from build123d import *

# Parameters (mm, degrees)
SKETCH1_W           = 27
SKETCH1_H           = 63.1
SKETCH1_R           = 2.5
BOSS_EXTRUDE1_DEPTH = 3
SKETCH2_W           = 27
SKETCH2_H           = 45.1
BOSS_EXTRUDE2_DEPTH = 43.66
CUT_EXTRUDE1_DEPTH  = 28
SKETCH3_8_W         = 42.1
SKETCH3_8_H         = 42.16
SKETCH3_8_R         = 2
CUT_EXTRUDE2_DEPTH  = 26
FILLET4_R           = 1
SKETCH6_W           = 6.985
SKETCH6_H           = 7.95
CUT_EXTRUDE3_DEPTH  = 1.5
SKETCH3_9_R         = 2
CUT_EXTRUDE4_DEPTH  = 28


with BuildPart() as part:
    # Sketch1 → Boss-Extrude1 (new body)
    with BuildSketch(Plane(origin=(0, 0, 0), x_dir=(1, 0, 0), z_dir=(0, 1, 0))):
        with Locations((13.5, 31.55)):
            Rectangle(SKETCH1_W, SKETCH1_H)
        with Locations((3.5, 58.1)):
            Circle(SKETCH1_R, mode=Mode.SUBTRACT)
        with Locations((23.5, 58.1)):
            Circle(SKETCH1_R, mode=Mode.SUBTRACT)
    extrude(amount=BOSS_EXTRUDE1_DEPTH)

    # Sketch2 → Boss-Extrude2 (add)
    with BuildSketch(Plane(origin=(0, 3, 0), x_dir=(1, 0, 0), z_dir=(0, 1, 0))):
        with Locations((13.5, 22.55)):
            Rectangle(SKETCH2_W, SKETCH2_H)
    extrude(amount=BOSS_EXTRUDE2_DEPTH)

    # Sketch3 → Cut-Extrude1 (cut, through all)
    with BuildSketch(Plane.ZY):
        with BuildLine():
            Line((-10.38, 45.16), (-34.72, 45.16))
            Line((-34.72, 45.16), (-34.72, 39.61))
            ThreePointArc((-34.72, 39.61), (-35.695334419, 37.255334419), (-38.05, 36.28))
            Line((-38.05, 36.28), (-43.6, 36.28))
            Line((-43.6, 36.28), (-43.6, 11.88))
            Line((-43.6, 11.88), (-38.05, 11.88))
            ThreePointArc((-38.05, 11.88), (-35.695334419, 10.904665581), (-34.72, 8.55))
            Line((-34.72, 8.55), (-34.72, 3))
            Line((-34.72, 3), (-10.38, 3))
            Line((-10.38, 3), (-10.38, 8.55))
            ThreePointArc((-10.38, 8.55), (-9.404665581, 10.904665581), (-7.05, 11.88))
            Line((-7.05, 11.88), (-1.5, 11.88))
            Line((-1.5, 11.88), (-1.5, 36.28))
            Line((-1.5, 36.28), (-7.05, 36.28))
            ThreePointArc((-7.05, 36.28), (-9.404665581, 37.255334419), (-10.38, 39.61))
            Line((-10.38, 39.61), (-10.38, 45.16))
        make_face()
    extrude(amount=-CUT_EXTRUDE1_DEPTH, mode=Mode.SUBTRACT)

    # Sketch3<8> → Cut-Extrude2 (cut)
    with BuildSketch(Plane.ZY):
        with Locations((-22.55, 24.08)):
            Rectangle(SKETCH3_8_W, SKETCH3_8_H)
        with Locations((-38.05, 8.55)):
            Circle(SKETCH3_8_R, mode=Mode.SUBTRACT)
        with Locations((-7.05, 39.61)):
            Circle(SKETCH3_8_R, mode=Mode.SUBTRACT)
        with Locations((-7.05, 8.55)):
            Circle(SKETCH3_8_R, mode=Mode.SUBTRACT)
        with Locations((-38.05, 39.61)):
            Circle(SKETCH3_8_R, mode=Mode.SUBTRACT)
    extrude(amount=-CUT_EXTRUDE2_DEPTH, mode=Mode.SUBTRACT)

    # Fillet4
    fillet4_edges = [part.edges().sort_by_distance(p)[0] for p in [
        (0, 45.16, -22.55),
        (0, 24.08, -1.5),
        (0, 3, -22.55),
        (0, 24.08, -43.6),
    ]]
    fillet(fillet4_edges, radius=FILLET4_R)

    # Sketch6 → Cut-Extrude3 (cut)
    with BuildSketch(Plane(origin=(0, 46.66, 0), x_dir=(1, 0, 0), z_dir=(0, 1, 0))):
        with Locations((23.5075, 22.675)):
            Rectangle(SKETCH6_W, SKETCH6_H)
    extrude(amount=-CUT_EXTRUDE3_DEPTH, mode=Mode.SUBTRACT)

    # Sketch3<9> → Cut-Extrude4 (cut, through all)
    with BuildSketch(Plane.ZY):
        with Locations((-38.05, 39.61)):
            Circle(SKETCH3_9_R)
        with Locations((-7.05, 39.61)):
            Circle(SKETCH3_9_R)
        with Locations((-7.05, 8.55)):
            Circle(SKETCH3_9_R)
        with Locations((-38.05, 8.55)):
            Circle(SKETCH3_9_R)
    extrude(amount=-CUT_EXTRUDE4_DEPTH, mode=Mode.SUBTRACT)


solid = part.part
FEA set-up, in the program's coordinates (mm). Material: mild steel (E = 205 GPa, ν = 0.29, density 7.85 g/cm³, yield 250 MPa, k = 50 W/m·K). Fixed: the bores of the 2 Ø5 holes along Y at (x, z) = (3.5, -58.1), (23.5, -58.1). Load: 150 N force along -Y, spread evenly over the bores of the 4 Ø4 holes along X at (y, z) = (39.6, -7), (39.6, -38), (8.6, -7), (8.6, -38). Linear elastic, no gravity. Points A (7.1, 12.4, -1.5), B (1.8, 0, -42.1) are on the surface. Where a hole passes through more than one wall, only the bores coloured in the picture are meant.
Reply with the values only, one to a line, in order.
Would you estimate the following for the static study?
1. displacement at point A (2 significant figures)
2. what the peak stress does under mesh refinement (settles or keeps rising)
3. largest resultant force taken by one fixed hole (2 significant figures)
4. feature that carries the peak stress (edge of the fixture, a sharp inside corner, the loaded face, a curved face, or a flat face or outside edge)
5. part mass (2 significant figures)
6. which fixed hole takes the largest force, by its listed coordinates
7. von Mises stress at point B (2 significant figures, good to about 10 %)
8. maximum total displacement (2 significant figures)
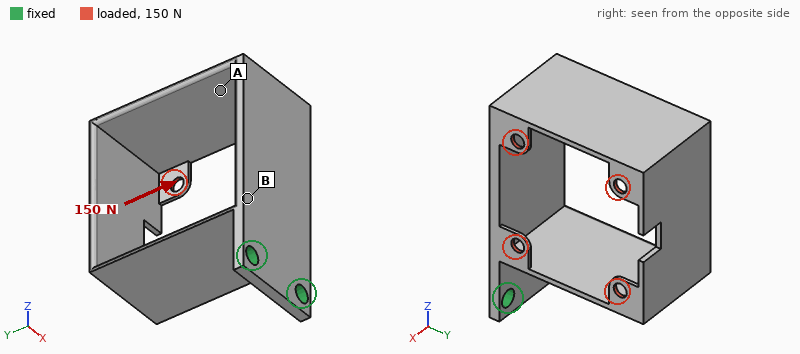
0.32 mm
keeps rising
170 N
edge of the fixture
81 g
(23.5, -58.1)
63 MPa
0.46 mm
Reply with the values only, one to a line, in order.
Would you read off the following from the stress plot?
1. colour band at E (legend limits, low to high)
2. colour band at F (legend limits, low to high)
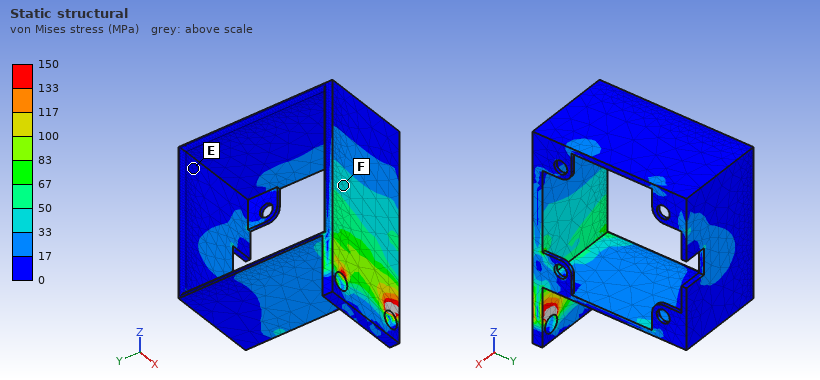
0 to 17 MPa
33 to 50 MPa
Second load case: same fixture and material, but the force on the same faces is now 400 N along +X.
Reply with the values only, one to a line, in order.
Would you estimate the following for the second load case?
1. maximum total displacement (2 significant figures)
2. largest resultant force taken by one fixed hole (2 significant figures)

0.44 mm
820 N
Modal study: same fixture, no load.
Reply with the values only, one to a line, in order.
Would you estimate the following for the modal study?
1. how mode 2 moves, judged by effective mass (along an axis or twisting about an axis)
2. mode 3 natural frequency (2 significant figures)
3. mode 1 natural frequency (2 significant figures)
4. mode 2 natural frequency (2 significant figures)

along X
960 Hz
340 Hz
780 Hz
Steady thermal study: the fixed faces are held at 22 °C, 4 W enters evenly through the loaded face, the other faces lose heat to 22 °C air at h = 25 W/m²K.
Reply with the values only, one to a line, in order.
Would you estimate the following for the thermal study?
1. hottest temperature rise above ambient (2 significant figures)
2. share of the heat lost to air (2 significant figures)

30 K
67 %
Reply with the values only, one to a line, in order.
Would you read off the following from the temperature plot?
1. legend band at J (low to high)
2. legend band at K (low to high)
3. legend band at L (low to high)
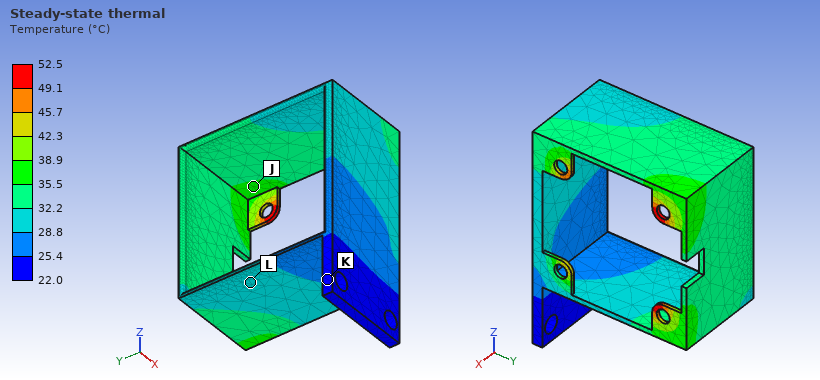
35.5 to 38.9 °C
22.0 to 25.4 °C
28.8 to 32.2 °C
